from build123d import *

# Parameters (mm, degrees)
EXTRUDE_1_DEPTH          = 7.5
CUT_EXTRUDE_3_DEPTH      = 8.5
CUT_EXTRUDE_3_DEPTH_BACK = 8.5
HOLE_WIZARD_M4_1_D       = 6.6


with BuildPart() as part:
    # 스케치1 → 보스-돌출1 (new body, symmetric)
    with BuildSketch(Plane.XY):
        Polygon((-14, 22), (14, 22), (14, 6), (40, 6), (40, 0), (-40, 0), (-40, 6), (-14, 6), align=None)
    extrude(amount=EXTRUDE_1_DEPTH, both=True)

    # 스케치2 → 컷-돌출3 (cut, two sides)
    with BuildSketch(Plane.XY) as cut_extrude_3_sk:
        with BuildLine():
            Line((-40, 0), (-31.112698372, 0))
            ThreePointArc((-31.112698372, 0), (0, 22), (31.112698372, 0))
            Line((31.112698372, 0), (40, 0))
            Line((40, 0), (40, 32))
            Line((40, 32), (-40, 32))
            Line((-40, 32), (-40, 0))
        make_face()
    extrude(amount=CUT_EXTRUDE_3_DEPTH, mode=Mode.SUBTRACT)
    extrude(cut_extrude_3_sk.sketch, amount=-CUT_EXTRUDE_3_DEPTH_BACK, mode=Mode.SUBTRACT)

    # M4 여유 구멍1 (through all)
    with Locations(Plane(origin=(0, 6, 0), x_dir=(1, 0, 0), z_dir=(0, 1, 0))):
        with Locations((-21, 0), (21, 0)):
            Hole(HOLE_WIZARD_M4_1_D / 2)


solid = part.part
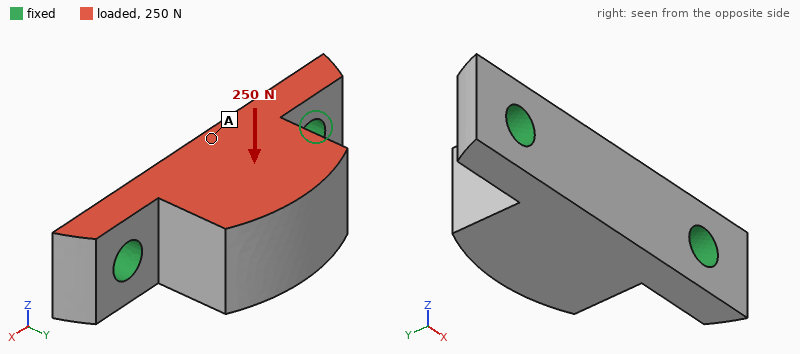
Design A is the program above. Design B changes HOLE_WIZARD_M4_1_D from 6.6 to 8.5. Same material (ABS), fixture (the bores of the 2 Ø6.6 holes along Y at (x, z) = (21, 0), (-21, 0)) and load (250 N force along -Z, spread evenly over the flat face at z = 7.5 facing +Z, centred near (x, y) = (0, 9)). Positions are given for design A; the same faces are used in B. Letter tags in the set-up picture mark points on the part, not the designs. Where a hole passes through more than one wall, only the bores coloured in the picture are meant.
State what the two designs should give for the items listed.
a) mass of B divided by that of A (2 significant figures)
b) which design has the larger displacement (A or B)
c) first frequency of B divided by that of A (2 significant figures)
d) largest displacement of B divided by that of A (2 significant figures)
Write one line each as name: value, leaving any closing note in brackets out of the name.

mass of B divided by that of A: 0.98
which design has the larger displacement: A
first frequency of B divided by that of A: 1.1
largest displacement of B divided by that of A: 0.80
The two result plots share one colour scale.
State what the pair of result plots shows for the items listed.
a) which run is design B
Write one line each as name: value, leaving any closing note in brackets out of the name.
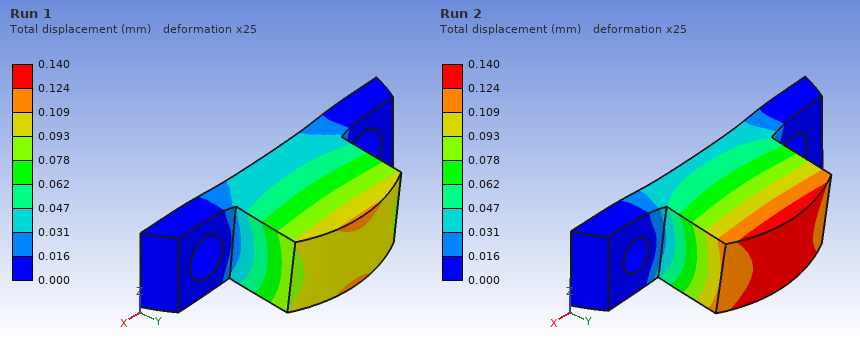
which run is design B: Run 1
